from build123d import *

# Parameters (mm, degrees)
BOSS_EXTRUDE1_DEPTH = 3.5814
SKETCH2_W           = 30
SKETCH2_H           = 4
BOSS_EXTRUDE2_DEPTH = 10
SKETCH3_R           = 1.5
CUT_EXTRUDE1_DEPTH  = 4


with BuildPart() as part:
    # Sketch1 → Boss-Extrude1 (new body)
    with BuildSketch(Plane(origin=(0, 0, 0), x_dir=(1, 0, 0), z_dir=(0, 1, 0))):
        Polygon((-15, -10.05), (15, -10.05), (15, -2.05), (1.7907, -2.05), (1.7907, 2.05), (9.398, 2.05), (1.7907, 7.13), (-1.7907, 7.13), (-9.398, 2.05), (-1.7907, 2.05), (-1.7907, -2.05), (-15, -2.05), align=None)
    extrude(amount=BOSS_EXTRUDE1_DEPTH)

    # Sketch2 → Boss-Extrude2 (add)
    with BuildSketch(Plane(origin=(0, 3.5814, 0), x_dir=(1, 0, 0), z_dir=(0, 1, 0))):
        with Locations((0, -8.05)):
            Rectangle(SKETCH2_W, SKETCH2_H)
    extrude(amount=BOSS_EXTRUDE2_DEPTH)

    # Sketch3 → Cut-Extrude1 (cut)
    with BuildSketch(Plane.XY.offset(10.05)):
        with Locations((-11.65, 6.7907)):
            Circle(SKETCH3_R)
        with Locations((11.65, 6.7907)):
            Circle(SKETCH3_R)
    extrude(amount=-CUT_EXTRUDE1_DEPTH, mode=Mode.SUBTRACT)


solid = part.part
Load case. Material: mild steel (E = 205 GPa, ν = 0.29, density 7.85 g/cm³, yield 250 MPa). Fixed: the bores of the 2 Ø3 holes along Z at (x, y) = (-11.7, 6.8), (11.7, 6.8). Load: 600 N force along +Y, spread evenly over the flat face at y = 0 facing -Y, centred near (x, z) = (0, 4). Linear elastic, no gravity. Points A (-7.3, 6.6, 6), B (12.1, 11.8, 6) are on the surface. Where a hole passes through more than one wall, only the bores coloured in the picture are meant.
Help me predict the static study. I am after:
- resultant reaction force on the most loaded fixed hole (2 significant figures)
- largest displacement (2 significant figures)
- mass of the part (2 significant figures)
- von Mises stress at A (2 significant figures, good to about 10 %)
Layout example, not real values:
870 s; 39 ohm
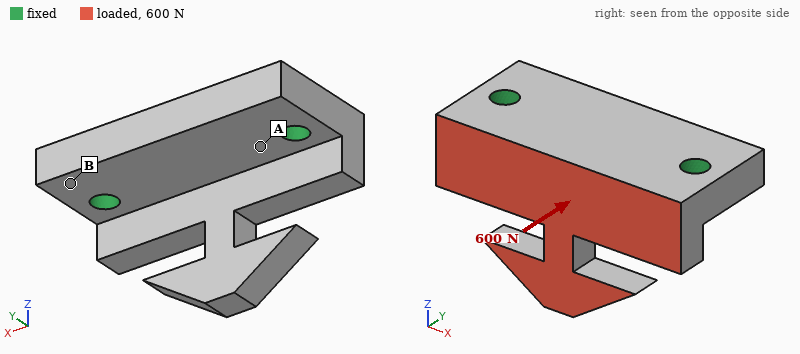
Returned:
300 N; 27 µm; 18 g; 27 MPa
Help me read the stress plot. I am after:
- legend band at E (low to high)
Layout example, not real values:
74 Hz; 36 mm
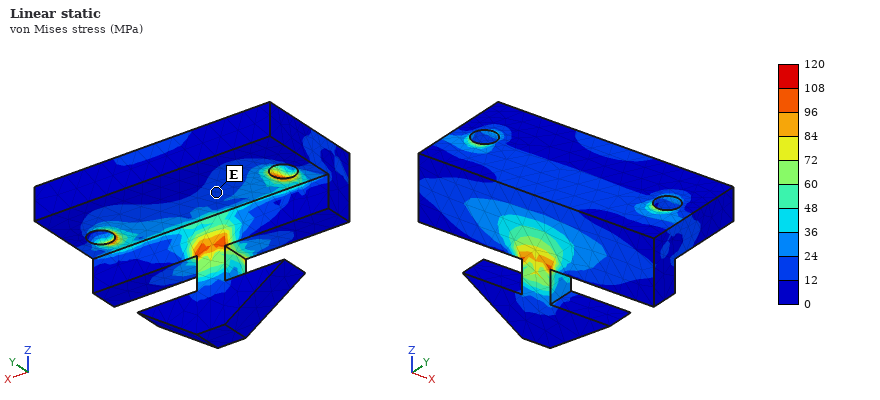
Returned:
12 to 24 MPa
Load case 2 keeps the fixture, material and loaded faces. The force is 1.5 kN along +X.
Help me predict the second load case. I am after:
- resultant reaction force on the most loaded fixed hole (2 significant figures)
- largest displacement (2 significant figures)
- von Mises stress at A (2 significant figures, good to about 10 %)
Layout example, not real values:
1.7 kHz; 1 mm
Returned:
880 N; 35 µm; 25 MPa
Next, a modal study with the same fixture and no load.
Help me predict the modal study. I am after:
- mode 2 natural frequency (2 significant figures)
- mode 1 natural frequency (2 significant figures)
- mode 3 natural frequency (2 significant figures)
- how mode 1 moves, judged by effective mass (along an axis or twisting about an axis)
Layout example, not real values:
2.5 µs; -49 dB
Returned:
13 kHz; 10 kHz; 17 kHz; along Y
